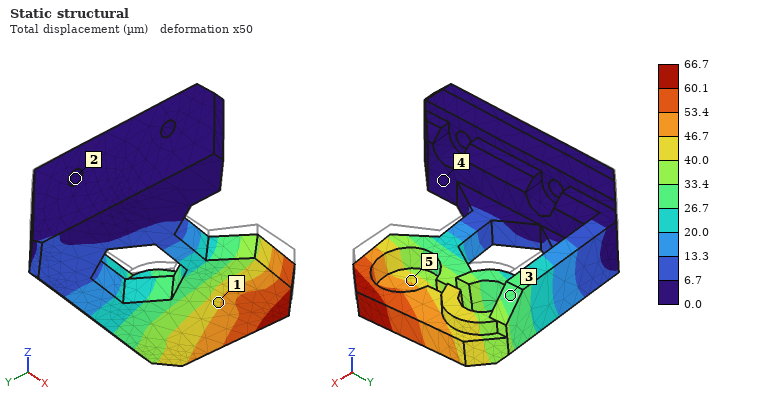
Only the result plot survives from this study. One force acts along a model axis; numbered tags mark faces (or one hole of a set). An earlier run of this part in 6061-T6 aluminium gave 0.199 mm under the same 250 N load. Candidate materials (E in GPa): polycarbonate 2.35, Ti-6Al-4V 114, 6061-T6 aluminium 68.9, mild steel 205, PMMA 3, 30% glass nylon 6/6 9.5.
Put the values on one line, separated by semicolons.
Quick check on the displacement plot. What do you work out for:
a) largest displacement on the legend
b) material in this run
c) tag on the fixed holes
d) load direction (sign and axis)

66.7 µm; mild steel; 2; -Z
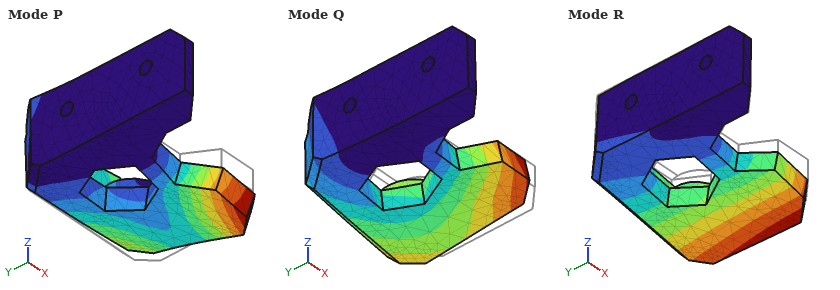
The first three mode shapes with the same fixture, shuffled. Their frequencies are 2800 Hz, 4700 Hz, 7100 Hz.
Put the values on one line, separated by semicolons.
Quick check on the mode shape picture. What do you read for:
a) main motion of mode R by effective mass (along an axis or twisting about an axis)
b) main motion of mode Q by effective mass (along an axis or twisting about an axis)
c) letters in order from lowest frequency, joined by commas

along Z; along Y; R, Q, P
